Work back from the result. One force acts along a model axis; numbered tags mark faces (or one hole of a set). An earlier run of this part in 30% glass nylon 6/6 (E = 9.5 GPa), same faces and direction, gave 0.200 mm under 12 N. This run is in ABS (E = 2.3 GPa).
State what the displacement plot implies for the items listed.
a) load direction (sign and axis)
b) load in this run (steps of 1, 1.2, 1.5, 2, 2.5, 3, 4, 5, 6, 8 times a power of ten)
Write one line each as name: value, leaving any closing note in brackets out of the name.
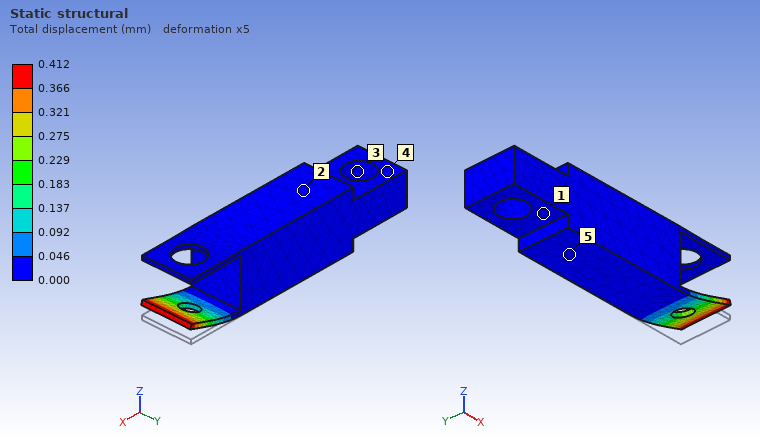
load direction: +Z
load in this run: 6 N
